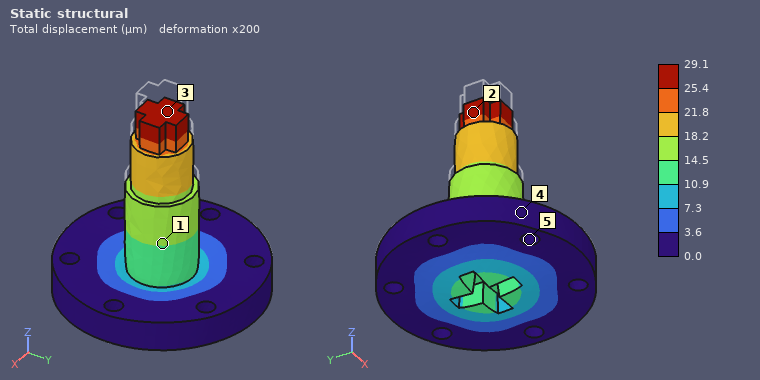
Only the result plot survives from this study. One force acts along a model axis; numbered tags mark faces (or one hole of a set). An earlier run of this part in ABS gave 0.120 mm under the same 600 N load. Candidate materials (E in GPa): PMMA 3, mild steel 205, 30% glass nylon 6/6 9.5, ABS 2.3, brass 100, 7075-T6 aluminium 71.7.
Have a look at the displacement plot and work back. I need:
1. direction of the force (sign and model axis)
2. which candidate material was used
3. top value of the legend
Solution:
-Z
30% glass nylon 6/6
29.1 µm
